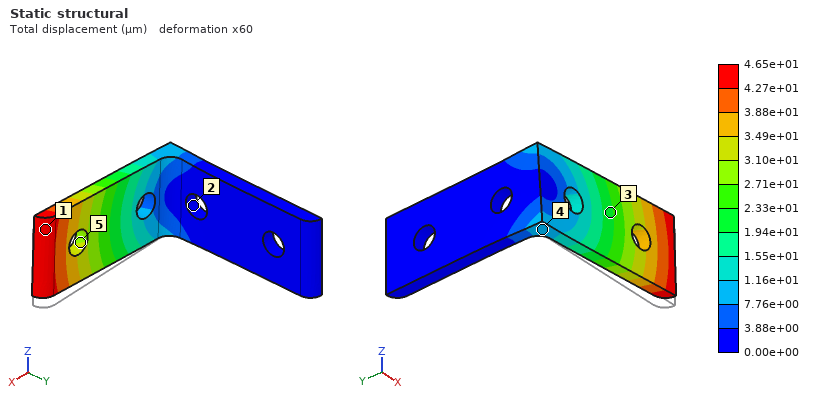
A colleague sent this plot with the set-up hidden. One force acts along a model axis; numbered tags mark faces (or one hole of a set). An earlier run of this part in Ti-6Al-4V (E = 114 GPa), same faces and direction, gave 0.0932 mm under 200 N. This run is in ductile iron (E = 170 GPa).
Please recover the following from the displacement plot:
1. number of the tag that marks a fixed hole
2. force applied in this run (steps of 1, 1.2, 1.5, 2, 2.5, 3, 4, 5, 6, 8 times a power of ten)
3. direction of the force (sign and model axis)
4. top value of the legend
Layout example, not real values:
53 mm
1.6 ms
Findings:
2
150 N
+Z
4.65e+01 µm
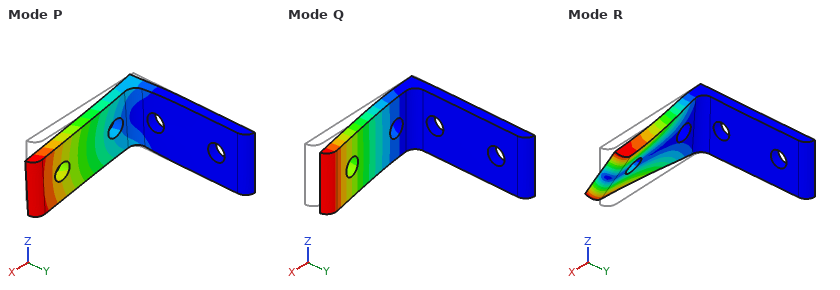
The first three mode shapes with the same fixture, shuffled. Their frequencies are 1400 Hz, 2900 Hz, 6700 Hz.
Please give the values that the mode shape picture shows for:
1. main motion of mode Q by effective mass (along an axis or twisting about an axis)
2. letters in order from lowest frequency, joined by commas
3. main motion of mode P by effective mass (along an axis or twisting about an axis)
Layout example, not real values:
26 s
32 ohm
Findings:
along Y
Q, P, R
along Z
